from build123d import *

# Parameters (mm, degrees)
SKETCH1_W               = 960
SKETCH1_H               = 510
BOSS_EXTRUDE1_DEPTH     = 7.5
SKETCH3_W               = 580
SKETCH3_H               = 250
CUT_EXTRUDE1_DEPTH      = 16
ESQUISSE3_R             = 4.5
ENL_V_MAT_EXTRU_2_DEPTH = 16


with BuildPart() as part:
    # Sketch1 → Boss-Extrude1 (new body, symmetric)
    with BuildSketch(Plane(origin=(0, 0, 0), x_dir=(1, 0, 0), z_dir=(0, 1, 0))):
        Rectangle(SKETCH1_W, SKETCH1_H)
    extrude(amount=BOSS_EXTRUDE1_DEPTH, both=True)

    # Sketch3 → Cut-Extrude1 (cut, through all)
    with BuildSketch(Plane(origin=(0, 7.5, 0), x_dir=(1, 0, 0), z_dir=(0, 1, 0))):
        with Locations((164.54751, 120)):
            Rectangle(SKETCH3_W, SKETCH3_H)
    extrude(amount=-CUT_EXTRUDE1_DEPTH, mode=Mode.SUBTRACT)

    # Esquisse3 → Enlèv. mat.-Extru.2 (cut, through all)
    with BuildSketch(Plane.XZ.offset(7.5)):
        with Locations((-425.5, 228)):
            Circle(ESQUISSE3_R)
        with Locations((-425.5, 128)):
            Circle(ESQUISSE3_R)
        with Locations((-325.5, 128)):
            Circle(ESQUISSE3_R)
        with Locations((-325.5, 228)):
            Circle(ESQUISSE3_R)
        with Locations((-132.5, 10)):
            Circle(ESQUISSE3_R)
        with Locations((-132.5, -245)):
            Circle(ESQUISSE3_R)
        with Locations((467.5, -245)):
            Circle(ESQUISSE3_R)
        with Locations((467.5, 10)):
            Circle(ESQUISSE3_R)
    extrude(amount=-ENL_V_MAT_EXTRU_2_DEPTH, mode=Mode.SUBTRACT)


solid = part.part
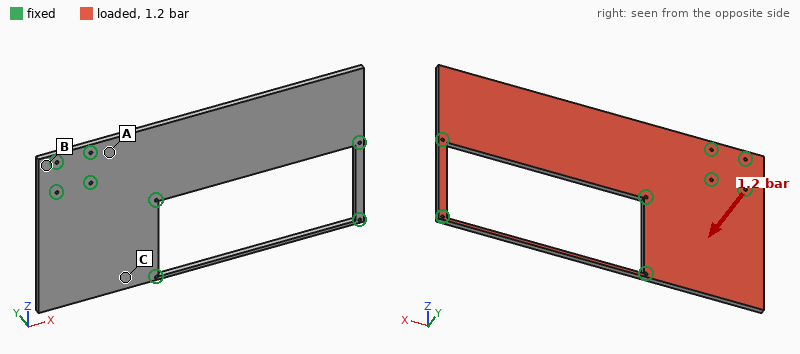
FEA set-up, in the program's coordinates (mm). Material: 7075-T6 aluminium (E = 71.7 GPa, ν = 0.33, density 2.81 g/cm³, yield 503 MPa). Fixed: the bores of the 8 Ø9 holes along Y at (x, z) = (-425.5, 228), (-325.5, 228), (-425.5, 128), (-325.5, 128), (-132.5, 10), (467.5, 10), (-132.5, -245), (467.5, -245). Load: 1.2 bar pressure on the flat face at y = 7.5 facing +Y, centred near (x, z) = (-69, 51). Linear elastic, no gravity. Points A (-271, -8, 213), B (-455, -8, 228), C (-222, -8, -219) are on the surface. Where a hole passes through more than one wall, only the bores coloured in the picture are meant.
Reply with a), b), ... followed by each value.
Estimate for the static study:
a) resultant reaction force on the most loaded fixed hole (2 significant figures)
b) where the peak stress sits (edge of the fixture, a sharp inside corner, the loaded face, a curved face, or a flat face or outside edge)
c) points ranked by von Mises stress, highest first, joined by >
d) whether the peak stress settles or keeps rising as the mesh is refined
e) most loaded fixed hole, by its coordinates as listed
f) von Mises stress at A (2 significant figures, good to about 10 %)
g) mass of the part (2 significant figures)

a) 13 kN
b) edge of the fixture
c) A > C > B
d) keeps rising
e) (-132.5, 10)
f) 90 MPa
g) 15 kg
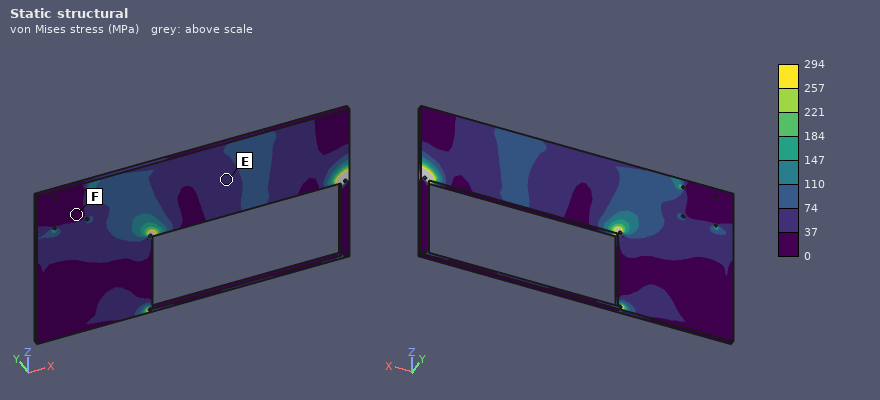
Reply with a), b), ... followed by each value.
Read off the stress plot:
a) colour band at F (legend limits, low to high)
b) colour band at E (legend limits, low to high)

a) 0 to 37 MPa
b) 37 to 74 MPa
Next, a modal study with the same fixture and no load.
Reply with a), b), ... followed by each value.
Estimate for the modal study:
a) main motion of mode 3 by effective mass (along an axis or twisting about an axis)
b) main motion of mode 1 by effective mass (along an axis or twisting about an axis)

a) along Y
b) along Y
